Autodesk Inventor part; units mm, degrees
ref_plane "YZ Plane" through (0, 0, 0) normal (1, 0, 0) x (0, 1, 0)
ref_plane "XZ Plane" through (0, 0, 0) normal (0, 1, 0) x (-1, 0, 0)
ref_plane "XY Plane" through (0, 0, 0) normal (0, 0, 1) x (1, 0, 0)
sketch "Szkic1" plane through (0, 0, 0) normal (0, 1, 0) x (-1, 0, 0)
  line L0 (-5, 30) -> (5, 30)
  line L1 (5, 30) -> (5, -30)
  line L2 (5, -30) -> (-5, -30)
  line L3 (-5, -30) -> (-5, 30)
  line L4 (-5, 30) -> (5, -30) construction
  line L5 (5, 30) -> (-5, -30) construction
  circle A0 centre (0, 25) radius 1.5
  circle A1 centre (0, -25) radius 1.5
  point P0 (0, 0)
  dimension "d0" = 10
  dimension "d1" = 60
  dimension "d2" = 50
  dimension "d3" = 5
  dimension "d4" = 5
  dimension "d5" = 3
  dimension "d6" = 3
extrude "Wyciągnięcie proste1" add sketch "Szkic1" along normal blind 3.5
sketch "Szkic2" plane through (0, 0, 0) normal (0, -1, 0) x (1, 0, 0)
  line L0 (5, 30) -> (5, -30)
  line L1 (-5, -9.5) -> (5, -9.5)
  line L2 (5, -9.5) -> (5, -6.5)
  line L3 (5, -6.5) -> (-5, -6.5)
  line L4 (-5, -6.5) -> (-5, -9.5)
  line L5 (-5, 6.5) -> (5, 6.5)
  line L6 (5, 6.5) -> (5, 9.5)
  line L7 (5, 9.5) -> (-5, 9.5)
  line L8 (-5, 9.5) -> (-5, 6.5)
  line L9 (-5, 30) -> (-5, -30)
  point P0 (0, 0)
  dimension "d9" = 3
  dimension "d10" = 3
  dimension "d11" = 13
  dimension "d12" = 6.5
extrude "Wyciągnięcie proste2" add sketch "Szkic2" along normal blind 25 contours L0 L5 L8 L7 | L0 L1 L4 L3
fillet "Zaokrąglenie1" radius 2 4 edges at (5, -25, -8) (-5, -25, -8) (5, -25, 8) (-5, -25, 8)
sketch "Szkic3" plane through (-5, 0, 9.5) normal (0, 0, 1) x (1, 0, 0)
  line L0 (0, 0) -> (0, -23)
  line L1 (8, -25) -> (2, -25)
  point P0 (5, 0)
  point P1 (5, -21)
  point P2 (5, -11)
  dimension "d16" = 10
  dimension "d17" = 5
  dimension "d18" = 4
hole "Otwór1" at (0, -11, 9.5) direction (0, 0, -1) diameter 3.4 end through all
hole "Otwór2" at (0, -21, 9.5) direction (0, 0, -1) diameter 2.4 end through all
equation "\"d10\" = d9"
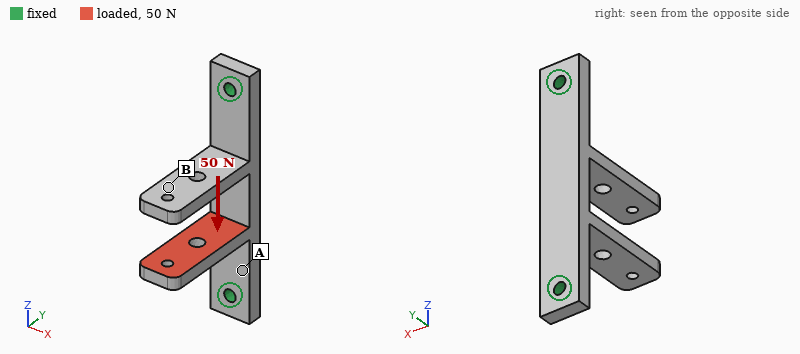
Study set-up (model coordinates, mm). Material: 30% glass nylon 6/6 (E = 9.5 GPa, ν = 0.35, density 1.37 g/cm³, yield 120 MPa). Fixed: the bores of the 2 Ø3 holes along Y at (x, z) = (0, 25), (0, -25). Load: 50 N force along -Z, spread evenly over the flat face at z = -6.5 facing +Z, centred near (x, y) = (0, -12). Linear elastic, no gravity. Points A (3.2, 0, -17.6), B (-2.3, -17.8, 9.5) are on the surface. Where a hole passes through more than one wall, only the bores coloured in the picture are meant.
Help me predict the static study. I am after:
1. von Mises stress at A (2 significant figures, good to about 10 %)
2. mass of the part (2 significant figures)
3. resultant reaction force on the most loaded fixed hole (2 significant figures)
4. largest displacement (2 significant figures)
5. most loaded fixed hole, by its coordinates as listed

7.2 MPa
4.7 g
37 N
0.71 mm
(0, -25)
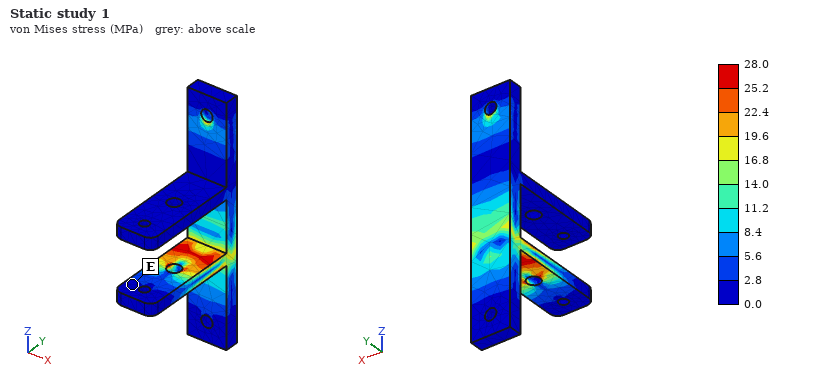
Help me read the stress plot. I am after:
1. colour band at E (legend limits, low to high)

0.0 to 2.8 MPa
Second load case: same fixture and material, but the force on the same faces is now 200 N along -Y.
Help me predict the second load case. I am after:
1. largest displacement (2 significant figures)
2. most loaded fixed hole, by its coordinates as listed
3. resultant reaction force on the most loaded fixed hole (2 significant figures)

0.79 mm
(0, -25)
140 N
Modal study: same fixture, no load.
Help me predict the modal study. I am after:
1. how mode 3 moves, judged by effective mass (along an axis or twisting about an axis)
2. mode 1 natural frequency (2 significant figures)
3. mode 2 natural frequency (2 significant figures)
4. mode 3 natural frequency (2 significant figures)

along Z
1500 Hz
1600 Hz
1800 Hz
